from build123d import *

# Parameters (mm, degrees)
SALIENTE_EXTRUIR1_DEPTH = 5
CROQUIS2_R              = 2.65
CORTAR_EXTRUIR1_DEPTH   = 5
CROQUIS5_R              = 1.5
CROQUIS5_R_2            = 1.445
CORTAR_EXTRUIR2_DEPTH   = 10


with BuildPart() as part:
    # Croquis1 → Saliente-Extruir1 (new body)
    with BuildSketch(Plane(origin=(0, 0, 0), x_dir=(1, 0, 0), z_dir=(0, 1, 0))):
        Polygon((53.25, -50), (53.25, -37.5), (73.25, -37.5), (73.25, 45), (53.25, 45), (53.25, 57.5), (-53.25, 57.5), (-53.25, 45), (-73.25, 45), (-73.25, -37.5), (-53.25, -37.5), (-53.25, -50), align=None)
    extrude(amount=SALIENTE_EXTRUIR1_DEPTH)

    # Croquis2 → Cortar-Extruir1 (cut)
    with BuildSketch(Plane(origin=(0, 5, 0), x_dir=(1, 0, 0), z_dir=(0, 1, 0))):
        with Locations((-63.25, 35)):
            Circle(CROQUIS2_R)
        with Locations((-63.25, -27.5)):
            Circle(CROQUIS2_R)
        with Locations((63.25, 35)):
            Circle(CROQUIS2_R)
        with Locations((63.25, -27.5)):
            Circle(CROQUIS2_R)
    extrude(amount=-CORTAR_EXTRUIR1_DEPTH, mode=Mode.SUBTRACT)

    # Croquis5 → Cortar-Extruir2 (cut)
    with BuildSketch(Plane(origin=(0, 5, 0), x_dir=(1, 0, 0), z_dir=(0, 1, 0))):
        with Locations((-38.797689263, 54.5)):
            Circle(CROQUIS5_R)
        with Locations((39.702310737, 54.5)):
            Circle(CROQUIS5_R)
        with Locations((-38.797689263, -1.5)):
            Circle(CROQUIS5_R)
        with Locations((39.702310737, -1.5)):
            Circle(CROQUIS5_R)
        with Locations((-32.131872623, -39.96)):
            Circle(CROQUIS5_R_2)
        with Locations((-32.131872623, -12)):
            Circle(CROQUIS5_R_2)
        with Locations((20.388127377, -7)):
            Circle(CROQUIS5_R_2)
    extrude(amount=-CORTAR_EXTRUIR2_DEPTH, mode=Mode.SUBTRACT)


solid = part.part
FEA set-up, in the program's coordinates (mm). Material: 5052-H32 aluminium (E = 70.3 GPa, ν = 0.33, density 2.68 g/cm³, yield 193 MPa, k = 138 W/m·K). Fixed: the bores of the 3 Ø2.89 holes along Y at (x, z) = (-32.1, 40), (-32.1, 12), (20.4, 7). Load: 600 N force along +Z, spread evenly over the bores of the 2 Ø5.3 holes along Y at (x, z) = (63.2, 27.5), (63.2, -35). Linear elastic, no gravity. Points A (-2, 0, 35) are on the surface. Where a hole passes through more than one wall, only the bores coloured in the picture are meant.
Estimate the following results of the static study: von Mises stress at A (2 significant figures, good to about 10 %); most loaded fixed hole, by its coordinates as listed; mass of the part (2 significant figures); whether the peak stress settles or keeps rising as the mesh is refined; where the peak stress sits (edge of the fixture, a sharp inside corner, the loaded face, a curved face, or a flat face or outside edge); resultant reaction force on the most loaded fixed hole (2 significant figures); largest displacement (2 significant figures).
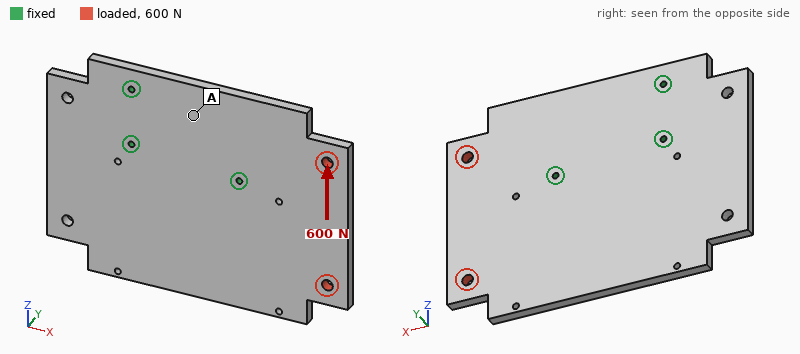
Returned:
2.0 MPa
(20.4, 7)
200 g
keeps rising
edge of the fixture
910 N
10 µm
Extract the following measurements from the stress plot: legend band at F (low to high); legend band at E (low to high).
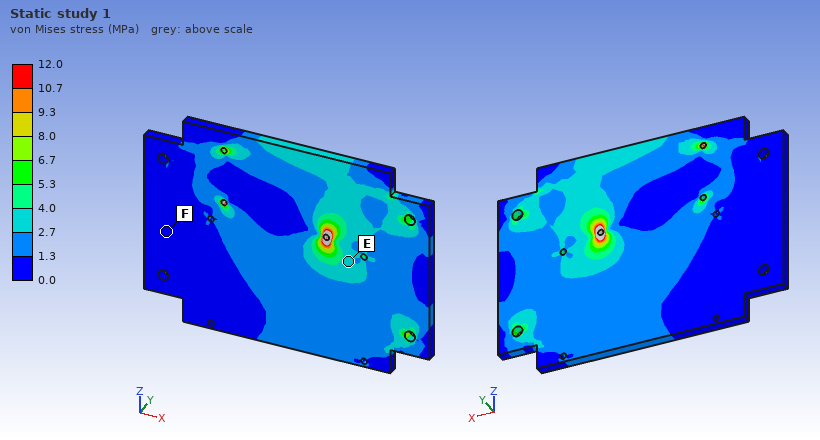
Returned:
0.0 to 1.3 MPa
2.7 to 4.0 MPa
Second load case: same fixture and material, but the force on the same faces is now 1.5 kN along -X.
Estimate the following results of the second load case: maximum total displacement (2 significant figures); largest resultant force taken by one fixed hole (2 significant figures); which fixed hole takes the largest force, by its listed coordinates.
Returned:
9.6 µm
1.0 kN
(20.4, 7)
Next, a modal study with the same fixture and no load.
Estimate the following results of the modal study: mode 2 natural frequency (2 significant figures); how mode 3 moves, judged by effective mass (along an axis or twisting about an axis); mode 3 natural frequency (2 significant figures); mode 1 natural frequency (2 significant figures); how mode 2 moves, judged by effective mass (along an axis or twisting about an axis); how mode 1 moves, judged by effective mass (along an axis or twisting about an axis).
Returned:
1000 Hz
along Y
1400 Hz
780 Hz
twisting about Z
along Y
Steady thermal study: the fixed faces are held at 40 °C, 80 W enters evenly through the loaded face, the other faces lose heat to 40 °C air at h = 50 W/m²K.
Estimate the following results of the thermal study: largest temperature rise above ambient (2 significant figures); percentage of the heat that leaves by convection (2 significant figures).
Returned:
81 K
41 %
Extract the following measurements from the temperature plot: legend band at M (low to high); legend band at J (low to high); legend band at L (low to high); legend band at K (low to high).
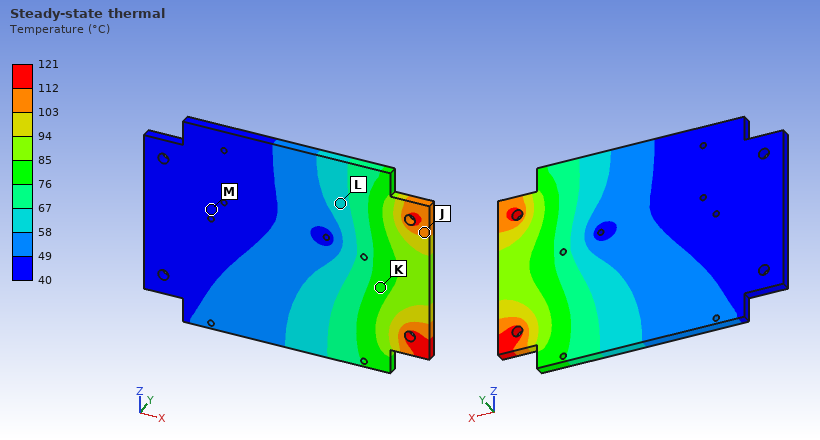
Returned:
40 to 49 °C
103 to 112 °C
58 to 67 °C
76 to 85 °C
